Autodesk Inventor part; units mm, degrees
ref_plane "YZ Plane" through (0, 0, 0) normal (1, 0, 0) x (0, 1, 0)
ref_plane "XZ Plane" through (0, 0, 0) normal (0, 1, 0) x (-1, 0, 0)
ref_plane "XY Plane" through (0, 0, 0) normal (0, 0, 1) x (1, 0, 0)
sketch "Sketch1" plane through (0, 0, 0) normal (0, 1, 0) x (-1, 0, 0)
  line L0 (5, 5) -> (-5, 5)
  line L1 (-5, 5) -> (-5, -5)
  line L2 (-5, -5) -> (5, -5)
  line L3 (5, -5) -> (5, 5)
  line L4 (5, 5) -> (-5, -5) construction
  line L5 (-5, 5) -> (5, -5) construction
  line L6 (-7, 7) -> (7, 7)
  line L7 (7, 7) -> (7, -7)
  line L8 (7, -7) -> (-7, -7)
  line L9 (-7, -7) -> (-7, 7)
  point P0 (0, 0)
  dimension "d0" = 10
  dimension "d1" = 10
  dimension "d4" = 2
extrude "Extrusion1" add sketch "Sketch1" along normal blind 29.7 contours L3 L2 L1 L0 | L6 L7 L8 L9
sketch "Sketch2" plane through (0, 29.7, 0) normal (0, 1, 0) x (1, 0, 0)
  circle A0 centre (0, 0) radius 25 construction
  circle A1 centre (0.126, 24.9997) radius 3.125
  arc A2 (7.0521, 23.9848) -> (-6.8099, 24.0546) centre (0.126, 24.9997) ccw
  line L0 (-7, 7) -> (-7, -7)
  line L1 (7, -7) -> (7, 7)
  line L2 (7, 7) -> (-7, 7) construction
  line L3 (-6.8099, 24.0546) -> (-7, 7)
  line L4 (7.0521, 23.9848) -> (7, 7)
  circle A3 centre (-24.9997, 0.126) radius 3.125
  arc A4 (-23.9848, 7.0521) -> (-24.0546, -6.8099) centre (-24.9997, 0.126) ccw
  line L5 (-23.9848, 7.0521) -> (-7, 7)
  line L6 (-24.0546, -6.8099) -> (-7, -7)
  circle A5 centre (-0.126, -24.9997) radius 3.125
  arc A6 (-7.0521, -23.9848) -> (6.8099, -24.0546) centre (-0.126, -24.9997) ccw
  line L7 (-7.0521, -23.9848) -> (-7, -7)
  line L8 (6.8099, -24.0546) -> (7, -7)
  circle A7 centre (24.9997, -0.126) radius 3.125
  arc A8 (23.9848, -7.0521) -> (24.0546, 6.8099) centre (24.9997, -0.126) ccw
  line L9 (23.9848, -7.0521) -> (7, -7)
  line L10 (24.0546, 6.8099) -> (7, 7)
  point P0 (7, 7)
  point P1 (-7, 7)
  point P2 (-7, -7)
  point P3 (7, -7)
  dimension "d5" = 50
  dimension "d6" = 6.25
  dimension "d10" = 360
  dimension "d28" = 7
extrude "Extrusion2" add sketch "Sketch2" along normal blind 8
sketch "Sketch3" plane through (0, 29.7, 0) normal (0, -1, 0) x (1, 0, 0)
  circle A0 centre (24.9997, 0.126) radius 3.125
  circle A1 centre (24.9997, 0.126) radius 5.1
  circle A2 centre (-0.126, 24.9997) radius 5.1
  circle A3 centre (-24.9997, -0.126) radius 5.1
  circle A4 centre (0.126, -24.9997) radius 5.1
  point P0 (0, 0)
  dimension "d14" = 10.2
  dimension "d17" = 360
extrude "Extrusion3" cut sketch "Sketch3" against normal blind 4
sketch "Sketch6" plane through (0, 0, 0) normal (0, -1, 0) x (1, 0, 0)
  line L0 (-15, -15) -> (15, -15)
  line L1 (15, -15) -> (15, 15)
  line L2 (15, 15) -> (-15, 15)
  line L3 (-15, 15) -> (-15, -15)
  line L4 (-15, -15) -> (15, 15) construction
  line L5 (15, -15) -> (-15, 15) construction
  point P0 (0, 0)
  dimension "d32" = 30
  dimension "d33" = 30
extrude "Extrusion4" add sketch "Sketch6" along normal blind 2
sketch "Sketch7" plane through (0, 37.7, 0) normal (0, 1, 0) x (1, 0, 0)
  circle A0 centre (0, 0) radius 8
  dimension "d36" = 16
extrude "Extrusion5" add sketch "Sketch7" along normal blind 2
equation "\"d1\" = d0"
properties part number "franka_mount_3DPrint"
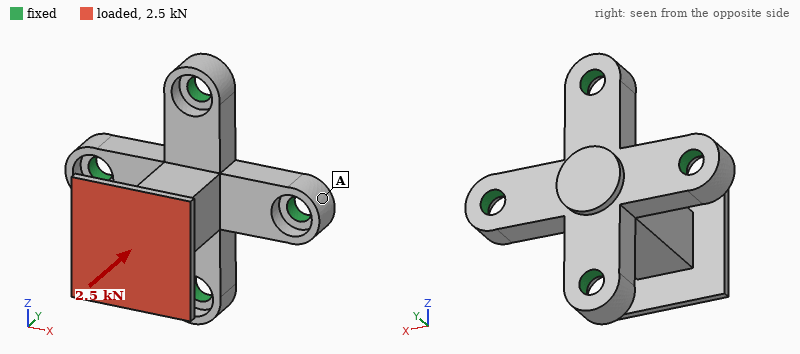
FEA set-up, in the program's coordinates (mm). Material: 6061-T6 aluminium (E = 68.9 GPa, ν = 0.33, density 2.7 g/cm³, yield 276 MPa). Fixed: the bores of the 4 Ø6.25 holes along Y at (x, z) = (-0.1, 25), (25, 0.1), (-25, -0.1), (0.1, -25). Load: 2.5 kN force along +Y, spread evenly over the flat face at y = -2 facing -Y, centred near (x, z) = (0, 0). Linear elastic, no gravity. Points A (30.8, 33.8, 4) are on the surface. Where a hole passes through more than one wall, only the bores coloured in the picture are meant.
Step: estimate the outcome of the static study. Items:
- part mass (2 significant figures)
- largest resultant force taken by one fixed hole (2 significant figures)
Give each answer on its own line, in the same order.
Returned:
49 g
850 N
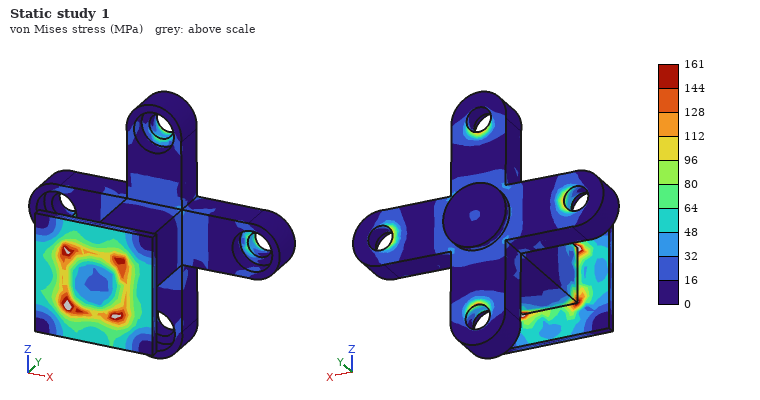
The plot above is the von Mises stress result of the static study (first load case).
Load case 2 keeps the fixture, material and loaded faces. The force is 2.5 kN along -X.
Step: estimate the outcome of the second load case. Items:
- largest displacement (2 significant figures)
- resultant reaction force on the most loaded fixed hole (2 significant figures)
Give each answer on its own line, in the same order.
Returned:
0.33 mm
2.6 kN
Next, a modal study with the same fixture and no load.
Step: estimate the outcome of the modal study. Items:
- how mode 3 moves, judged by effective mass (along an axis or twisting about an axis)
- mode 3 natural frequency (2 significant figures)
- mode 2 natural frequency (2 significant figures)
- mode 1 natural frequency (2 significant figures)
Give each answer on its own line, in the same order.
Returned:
along Y
10 kHz
5000 Hz
5000 Hz
